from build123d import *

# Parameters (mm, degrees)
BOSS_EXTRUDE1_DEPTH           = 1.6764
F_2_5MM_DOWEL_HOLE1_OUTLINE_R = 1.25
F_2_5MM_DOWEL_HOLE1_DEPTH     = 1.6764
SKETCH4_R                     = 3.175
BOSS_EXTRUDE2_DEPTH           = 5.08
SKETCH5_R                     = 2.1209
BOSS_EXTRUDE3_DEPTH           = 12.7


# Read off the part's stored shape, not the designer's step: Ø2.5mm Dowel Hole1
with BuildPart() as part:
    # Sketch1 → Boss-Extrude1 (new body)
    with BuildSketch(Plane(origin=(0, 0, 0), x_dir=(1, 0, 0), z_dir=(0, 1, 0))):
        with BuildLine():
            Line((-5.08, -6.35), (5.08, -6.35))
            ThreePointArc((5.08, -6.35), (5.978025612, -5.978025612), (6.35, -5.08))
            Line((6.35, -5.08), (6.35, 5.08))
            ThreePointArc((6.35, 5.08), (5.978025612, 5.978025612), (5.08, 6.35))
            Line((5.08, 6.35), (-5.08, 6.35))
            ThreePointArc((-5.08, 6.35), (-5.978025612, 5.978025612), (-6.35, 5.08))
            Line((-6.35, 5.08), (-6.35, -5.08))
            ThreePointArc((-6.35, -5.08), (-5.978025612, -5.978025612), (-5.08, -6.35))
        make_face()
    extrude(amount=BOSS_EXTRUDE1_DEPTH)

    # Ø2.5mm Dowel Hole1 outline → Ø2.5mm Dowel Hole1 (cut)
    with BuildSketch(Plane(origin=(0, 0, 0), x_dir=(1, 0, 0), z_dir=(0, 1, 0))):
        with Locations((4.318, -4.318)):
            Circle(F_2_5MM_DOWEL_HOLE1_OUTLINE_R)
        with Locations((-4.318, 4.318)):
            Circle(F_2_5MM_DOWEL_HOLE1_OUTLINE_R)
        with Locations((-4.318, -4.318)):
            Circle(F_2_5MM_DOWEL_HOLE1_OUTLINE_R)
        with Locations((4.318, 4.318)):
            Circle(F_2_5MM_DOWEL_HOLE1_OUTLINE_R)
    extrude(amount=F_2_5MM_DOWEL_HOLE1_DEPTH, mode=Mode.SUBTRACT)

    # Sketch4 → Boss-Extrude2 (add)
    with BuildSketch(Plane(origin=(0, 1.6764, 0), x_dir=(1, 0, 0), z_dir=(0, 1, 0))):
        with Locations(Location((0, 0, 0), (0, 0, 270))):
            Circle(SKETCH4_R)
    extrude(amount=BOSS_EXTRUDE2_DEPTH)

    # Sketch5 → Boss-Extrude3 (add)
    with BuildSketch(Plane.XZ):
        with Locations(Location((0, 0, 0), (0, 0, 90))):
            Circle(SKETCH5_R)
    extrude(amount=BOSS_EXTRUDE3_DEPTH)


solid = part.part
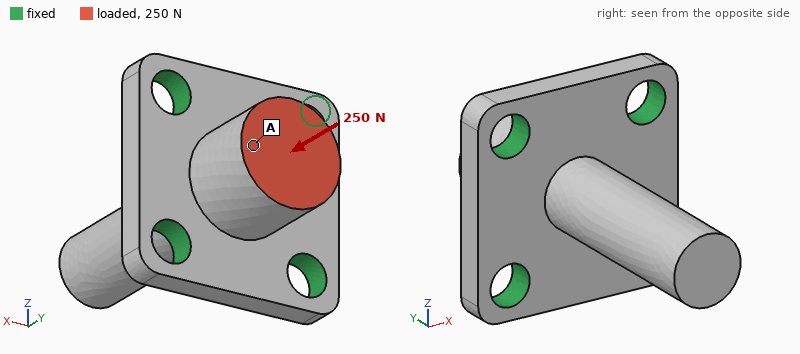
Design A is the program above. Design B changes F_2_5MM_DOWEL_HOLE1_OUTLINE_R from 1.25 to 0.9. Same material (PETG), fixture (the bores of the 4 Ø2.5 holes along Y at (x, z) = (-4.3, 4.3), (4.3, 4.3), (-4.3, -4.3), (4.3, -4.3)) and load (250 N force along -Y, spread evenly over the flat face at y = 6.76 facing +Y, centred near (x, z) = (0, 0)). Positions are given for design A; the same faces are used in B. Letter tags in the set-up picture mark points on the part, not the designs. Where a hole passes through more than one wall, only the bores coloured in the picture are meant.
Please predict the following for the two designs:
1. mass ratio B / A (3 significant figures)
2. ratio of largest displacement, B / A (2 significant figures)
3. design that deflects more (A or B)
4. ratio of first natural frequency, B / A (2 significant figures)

1.03
1.2
B
0.98
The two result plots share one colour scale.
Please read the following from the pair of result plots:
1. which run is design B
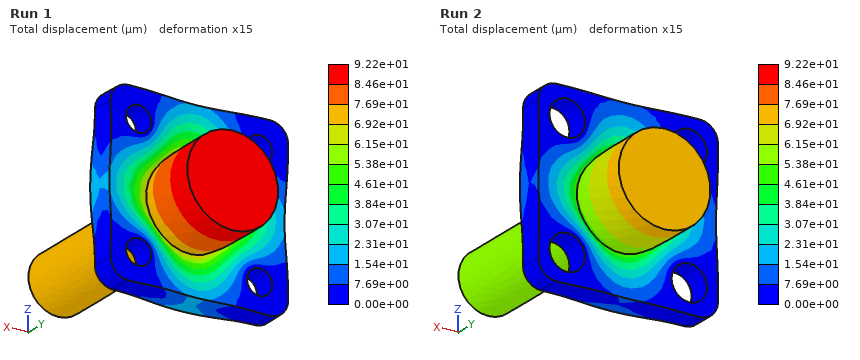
Run 1
